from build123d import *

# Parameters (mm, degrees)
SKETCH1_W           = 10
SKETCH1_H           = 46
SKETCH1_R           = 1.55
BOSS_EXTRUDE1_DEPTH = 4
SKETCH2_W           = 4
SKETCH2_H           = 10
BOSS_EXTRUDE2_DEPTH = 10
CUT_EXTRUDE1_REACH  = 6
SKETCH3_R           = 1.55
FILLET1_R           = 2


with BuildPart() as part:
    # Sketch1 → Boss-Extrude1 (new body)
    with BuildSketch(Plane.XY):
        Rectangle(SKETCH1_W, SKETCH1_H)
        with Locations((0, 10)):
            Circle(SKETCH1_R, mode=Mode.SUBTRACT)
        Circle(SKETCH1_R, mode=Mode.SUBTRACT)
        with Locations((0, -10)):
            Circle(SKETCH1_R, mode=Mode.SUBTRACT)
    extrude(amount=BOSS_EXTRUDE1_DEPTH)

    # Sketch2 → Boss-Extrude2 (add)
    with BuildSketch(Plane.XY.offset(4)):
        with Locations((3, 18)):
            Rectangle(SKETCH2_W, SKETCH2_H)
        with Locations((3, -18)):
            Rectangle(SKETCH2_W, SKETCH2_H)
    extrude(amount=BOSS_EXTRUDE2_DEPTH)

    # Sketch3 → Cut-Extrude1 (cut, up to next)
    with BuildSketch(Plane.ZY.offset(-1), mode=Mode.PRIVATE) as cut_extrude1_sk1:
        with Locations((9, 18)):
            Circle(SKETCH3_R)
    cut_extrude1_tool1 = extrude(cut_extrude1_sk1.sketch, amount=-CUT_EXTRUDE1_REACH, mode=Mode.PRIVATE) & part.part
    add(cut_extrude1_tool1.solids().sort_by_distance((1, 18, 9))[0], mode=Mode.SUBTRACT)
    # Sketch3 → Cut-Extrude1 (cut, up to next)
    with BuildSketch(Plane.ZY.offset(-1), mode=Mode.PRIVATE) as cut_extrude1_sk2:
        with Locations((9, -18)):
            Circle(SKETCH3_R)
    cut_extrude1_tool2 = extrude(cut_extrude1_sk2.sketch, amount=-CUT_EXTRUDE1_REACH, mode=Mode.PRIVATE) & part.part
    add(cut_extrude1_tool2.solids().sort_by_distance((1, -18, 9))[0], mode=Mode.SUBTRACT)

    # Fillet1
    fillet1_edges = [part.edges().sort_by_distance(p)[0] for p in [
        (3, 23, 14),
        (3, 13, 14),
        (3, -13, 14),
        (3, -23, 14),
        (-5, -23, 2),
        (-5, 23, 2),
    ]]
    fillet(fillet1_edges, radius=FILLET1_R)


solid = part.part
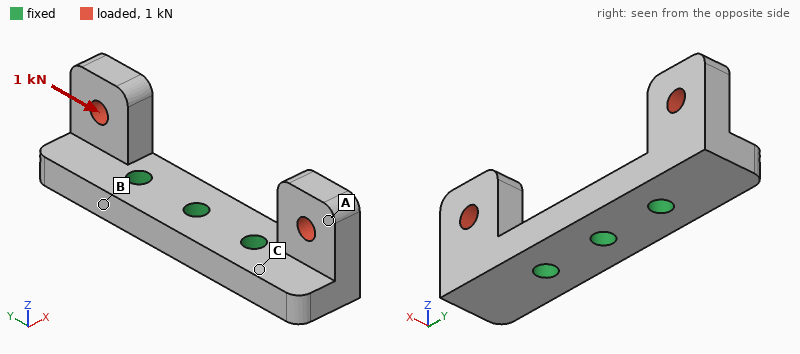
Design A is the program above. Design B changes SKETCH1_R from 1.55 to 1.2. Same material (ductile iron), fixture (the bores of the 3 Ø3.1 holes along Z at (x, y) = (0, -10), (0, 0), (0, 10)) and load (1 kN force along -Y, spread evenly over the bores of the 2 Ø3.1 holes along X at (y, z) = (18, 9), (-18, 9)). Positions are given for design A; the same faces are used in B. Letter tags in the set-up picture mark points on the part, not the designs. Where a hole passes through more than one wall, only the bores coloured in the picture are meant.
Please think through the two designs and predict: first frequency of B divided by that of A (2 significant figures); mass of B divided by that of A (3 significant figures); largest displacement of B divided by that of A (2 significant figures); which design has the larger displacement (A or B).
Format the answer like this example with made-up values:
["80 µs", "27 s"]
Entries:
["0.94", "1.01", "1.1", "B"]
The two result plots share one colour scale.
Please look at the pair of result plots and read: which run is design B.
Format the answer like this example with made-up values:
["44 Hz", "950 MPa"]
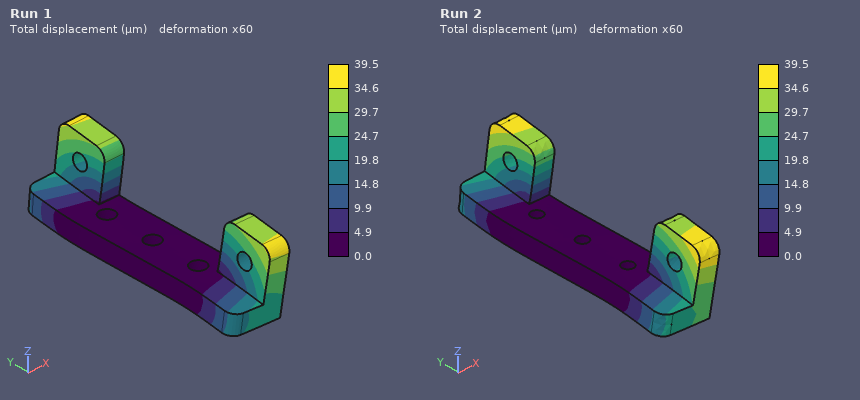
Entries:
["Run 2"]
